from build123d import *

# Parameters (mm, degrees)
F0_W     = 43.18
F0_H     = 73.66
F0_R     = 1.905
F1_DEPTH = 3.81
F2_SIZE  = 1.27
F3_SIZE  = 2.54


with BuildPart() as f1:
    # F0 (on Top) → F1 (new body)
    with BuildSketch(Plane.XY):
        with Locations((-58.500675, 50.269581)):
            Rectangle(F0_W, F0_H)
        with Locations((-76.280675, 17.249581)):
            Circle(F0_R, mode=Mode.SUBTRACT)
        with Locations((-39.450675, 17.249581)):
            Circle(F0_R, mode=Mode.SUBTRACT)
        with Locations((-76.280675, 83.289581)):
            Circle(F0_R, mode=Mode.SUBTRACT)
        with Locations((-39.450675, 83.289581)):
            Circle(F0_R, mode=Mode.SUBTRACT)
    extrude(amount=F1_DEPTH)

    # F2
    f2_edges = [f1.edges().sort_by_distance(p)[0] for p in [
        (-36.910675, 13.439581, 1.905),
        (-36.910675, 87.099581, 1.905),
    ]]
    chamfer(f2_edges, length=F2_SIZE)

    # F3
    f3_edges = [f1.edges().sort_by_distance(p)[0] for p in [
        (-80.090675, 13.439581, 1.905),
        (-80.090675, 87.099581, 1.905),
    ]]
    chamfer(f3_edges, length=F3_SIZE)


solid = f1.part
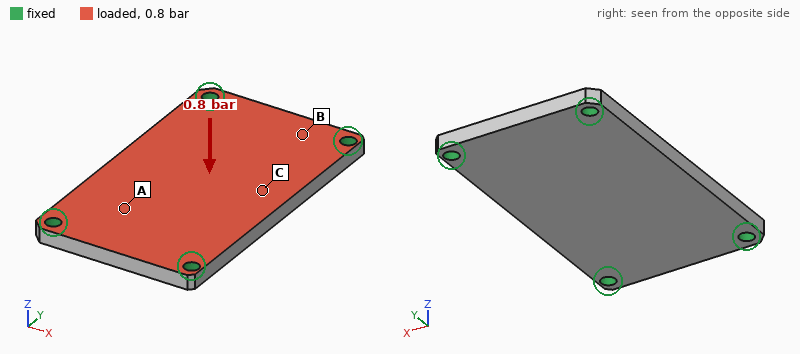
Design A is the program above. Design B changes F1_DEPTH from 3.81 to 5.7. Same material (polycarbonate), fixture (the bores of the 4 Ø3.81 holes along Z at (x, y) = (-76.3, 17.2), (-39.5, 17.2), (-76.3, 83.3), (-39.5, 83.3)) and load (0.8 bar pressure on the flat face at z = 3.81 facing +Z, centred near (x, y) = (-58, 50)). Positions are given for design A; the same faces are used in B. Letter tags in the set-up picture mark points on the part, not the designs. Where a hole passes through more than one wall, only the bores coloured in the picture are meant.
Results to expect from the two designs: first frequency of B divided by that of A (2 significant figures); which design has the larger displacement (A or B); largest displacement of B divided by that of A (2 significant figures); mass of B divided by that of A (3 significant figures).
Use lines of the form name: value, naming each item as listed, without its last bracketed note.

first frequency of B divided by that of A: 1.4
which design has the larger displacement: A
largest displacement of B divided by that of A: 0.33
mass of B divided by that of A: 1.50
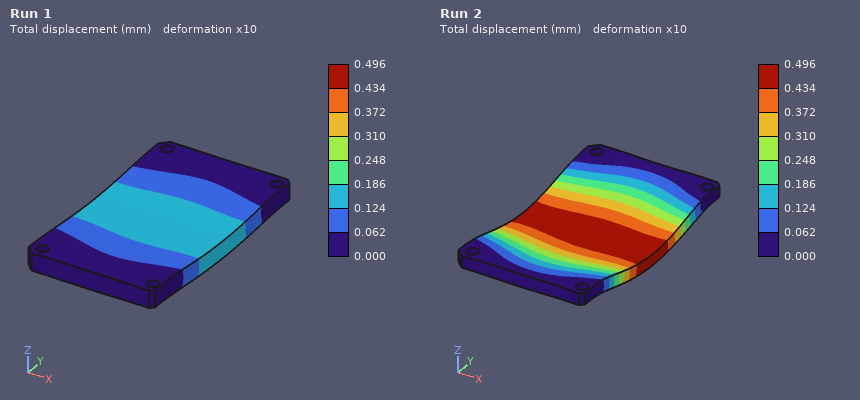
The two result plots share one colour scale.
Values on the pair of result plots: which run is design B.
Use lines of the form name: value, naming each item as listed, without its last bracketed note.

which run is design B: Run 1
